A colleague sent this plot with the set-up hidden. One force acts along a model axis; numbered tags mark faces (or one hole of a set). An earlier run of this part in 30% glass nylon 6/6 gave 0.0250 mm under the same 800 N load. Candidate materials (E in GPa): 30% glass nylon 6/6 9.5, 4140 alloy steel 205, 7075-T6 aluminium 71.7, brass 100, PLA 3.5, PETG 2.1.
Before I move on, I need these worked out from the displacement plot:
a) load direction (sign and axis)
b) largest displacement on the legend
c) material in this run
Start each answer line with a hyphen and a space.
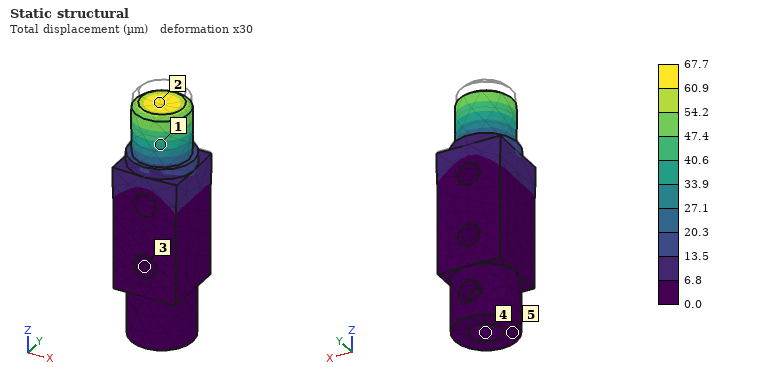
- -Z
- 67.7 µm
- PLA
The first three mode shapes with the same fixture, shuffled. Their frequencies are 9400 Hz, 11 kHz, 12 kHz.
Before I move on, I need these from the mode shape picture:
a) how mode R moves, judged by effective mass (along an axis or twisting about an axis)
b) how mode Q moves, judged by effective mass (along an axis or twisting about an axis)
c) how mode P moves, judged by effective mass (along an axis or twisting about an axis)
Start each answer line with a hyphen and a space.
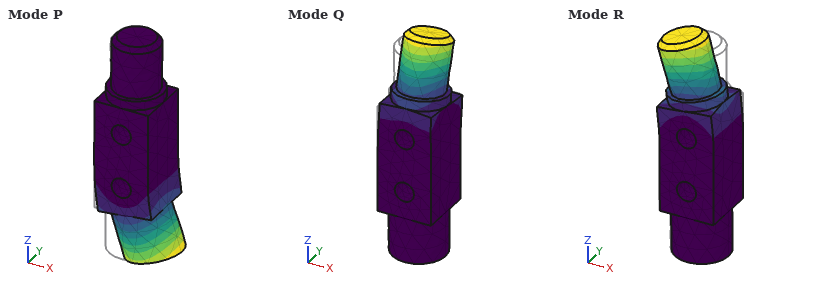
- along X
- along Y
- along X
